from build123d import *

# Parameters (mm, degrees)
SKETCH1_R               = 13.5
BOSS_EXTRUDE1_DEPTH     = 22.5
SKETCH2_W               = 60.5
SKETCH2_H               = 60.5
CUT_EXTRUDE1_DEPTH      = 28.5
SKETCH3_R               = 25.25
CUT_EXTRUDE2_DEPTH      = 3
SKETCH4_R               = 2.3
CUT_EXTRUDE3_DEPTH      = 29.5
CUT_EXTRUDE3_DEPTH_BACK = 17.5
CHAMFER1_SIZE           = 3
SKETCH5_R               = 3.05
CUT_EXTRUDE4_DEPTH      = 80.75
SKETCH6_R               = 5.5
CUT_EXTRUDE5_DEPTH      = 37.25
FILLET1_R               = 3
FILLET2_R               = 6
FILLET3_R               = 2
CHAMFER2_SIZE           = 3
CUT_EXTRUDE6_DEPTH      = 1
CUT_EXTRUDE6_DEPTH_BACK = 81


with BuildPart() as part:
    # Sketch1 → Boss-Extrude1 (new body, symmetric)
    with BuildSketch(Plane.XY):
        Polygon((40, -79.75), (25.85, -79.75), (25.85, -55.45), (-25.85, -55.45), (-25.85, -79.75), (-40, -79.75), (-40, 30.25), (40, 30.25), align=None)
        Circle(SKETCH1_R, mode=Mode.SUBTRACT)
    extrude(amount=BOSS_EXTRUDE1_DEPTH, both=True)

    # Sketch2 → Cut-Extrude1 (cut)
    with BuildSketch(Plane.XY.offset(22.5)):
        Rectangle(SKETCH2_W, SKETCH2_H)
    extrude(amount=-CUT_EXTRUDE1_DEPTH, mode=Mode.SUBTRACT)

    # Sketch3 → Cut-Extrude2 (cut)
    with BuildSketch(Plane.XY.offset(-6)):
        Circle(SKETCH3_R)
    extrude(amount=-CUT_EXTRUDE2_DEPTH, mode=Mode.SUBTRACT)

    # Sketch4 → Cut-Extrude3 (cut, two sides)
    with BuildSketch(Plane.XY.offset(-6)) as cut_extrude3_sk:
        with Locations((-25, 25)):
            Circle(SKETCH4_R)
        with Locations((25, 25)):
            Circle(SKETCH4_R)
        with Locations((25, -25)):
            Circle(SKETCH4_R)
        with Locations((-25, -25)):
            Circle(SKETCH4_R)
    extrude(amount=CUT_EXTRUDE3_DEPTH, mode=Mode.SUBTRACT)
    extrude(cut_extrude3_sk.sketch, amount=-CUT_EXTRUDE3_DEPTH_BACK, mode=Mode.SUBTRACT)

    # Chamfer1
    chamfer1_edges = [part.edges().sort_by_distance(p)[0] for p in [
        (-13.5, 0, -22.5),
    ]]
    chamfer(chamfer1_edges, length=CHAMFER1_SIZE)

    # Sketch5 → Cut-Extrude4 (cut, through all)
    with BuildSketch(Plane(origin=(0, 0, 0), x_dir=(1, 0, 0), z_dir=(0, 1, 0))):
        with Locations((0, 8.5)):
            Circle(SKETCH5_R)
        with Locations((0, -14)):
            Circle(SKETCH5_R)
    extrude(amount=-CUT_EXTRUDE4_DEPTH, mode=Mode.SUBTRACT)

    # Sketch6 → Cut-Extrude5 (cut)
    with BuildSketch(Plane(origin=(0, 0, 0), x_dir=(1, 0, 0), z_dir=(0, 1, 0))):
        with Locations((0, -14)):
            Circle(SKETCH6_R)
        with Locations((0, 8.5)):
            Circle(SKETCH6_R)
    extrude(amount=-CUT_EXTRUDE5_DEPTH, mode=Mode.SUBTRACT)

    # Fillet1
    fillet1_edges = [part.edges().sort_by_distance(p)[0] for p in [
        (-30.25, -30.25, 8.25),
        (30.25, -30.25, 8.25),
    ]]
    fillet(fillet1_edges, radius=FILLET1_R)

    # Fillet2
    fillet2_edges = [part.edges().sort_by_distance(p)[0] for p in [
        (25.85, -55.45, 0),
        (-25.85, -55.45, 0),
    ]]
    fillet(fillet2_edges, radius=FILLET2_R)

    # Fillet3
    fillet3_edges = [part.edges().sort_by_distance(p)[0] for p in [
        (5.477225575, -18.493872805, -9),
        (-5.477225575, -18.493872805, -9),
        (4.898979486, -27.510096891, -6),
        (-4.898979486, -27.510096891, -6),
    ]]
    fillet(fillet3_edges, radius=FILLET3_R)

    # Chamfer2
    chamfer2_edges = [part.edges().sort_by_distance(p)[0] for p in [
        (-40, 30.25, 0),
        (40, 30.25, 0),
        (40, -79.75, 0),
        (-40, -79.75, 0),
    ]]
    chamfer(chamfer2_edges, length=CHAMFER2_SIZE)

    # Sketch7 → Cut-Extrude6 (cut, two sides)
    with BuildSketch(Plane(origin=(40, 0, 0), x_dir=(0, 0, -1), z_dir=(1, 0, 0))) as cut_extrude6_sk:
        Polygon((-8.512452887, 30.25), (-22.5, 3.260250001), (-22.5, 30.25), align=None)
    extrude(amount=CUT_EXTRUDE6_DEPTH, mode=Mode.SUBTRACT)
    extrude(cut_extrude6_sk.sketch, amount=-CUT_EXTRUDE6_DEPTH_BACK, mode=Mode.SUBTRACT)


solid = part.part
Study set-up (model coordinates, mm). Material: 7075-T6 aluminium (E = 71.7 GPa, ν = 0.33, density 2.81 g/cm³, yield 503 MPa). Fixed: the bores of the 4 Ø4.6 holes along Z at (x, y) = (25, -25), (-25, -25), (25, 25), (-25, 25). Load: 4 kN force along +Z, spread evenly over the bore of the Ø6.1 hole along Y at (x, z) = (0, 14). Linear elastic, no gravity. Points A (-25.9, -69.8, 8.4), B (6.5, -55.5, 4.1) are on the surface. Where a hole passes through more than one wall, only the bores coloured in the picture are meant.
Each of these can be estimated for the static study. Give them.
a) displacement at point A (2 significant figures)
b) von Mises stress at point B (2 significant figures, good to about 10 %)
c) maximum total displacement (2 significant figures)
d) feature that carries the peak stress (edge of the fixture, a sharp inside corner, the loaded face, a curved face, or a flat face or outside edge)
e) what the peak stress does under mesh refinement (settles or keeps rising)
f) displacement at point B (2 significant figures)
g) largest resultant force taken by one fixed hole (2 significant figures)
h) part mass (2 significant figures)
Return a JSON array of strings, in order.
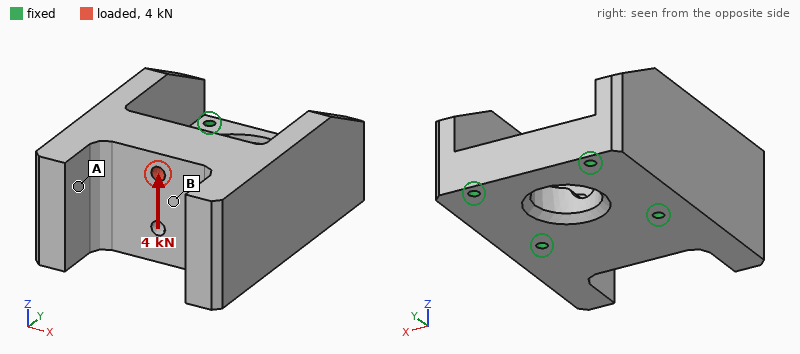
["13 µm", "8.6 MPa", "17 µm", "edge of the fixture", "keeps rising", "12 µm", "2.6 kN", "600 g"]
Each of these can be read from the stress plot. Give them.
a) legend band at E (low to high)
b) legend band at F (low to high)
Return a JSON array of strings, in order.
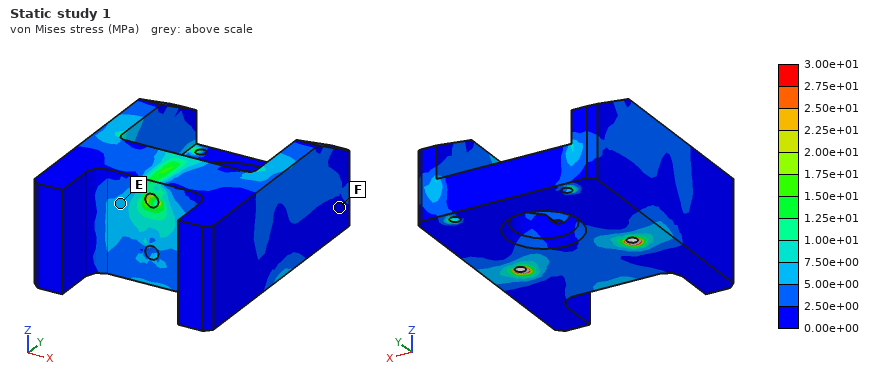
["5.00e+00 to 7.50e+00 MPa", "0.00e+00 to 2.50e+00 MPa"]
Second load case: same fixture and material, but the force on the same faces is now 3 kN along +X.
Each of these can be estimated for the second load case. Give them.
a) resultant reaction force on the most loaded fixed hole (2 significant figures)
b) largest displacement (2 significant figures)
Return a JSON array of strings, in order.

["2.3 kN", "8.8 µm"]
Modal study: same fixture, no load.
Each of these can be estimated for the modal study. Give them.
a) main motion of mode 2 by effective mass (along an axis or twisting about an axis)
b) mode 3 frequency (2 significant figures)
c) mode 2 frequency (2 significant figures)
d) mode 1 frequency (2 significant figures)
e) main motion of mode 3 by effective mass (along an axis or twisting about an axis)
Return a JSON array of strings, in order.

["along X", "7400 Hz", "5800 Hz", "4700 Hz", "along X"]
